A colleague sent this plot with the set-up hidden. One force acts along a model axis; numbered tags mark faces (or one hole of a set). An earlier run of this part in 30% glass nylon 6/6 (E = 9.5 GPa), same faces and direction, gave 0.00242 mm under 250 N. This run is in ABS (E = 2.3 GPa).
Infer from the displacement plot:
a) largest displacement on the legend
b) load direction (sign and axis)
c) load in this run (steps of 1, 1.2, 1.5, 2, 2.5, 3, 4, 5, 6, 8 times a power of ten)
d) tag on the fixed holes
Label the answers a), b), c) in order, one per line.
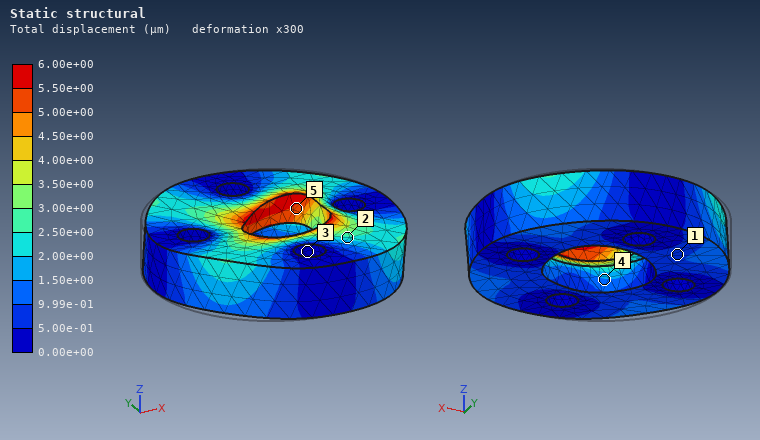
a) 6.00e+00 µm
b) +X
c) 150 N
d) 3
